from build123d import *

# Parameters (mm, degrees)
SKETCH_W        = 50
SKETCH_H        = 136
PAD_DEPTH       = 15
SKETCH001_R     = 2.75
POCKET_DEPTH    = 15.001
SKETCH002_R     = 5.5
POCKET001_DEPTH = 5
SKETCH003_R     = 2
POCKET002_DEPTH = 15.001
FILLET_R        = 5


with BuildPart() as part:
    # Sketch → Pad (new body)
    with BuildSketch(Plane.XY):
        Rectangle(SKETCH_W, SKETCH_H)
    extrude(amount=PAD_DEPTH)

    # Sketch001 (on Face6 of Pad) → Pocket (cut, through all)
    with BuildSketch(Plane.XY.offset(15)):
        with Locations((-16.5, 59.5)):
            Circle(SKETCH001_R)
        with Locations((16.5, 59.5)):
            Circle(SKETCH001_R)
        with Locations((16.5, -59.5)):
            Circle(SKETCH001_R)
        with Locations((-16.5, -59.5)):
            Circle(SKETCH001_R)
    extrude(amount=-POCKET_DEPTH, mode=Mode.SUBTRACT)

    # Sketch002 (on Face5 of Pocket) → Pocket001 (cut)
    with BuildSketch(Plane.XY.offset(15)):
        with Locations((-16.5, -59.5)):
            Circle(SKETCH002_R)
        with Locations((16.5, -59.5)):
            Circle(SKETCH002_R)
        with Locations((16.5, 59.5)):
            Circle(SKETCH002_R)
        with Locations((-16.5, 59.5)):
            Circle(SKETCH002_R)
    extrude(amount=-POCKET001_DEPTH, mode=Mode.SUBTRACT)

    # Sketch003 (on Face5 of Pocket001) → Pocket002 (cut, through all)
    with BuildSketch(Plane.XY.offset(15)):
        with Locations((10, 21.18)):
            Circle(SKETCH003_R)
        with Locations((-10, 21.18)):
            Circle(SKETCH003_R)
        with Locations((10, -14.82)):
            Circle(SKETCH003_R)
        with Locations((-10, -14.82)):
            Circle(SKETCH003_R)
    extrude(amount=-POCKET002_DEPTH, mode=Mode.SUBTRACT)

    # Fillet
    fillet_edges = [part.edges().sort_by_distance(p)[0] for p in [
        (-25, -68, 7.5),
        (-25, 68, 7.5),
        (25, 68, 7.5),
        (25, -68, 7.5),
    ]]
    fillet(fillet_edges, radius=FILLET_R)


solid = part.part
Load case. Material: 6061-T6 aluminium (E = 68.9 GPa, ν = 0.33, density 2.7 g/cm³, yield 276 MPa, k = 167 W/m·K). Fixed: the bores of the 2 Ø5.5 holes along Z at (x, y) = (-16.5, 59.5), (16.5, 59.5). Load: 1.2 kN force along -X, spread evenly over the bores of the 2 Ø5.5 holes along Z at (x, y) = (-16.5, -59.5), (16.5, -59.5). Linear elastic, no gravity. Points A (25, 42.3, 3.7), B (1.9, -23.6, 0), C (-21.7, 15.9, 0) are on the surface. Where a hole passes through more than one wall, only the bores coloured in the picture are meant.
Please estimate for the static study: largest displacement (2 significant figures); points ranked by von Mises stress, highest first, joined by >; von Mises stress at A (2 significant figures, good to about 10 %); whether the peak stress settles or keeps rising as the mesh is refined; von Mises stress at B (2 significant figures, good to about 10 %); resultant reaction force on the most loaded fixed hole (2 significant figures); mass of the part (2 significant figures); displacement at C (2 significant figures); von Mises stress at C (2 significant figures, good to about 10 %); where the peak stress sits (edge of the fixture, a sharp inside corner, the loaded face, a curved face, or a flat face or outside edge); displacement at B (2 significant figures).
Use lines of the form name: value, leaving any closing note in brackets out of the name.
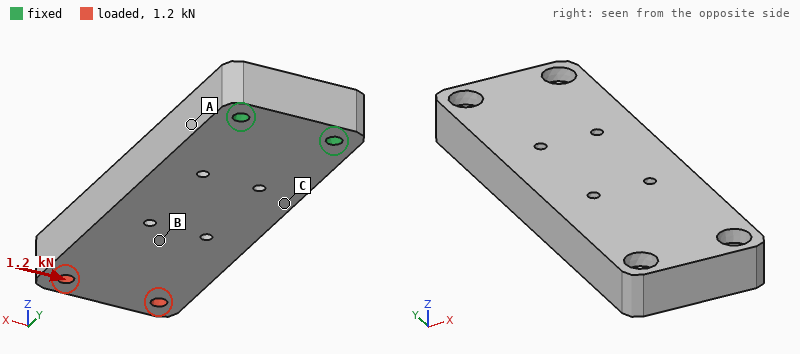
largest displacement: 96 µm
points ranked by von Mises stress, highest first, joined by >: A > C > B
von Mises stress at A: 20 MPa
whether the peak stress settles or keeps rising as the mesh is refined: keeps rising
von Mises stress at B: 5.5 MPa
resultant reaction force on the most loaded fixed hole: 4.1 kN
mass of the part: 260 g
displacement at C: 24 µm
von Mises stress at C: 13 MPa
where the peak stress sits: edge of the fixture
displacement at B: 52 µm
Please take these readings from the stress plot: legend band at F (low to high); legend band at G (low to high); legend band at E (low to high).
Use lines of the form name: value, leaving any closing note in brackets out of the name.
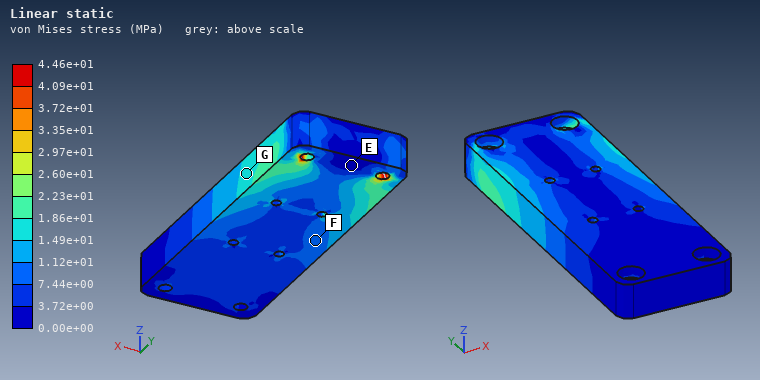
legend band at F: 7.44e+00 to 1.12e+01 MPa
legend band at G: 1.49e+01 to 1.86e+01 MPa
legend band at E: 0.00e+00 to 3.72e+00 MPa
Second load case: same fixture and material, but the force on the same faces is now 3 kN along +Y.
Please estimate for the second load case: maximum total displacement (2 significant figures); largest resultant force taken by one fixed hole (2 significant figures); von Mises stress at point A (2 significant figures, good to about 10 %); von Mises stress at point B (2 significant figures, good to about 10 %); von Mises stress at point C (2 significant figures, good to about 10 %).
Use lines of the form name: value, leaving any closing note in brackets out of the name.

maximum total displacement: 61 µm
largest resultant force taken by one fixed hole: 1.5 kN
von Mises stress at point A: 6.4 MPa
von Mises stress at point B: 8.3 MPa
von Mises stress at point C: 8.4 MPa
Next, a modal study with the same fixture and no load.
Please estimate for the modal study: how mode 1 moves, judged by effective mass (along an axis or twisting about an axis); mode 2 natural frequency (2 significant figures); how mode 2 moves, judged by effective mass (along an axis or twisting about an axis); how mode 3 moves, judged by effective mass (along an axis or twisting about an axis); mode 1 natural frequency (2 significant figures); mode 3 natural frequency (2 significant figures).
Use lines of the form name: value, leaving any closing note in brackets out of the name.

how mode 1 moves, judged by effective mass: along Z
mode 2 natural frequency: 2100 Hz
how mode 2 moves, judged by effective mass: along X
how mode 3 moves, judged by effective mass: twisting about Y
mode 1 natural frequency: 640 Hz
mode 3 natural frequency: 3300 Hz
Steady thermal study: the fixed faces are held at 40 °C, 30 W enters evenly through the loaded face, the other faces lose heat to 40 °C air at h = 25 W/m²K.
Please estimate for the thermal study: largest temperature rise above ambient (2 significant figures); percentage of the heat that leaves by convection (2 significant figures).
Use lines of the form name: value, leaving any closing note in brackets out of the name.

largest temperature rise above ambient: 28 K
percentage of the heat that leaves by convection: 22 %
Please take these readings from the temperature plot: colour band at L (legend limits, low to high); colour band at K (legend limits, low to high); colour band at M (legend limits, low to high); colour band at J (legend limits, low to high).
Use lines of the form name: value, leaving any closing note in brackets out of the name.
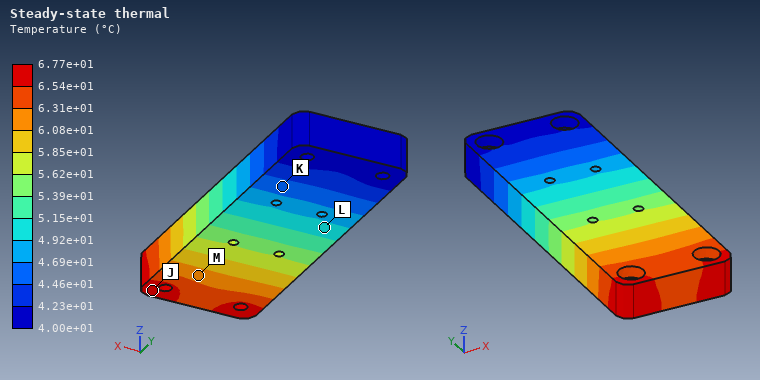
colour band at L: 4.92e+01 to 5.15e+01 °C
colour band at K: 4.46e+01 to 4.69e+01 °C
colour band at M: 6.08e+01 to 6.31e+01 °C
colour band at J: 6.54e+01 to 6.77e+01 °C
